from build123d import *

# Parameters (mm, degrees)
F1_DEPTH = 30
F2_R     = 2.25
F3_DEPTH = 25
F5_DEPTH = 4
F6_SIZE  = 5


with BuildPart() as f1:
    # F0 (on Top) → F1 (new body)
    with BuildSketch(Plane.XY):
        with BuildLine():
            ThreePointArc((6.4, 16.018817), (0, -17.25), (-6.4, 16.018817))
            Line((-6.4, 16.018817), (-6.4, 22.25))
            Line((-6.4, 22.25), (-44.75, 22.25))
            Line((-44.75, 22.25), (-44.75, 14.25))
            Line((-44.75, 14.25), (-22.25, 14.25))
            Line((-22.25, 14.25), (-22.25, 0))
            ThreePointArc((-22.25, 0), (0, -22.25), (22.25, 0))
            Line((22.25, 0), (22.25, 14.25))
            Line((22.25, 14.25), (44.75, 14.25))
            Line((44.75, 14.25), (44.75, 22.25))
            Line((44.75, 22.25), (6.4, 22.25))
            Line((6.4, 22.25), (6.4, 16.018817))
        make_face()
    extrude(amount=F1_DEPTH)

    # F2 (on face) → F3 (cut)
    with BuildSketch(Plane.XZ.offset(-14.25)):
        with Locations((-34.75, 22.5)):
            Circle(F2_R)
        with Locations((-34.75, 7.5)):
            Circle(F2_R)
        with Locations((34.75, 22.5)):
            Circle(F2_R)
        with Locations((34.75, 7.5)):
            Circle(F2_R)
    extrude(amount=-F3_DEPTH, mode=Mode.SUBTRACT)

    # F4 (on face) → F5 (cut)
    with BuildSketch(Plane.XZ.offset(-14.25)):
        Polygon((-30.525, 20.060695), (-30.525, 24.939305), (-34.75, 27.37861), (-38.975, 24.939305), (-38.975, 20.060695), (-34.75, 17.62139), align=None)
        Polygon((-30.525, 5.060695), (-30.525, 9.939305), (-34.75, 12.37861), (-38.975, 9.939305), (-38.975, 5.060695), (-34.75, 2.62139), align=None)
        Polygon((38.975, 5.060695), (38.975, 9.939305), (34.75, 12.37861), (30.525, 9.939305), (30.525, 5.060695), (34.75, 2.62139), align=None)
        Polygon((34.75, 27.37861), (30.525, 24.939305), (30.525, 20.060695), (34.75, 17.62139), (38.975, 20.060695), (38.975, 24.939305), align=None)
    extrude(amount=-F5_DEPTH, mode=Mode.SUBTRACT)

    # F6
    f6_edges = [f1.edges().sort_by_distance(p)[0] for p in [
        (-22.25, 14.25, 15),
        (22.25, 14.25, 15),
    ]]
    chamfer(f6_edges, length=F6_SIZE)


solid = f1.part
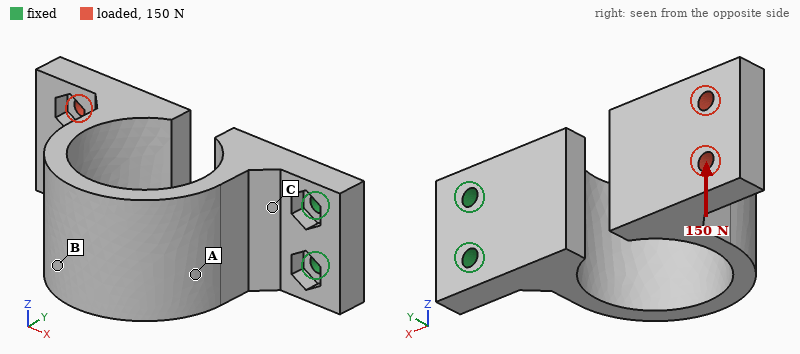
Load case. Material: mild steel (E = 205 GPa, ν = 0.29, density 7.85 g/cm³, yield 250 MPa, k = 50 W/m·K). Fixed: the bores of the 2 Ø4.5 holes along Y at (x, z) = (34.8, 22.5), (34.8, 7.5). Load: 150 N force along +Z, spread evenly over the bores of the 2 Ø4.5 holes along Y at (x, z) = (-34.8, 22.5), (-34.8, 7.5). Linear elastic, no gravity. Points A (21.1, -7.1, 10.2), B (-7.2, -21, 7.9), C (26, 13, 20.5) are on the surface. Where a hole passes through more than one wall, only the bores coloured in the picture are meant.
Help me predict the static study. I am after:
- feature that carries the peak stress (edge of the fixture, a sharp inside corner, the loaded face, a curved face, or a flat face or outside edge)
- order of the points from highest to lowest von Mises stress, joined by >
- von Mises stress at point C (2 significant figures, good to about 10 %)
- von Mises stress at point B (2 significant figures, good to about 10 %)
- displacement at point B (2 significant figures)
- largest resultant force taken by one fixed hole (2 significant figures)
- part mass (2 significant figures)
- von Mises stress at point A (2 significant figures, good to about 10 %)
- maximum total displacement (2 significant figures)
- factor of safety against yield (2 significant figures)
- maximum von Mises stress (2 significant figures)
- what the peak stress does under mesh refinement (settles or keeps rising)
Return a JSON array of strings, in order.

["a curved face", "A > B > C", "12 MPa", "29 MPa", "0.044 mm", "580 N", "260 g", "52 MPa", "0.22 mm", "3.9", "65 MPa", "settles"]
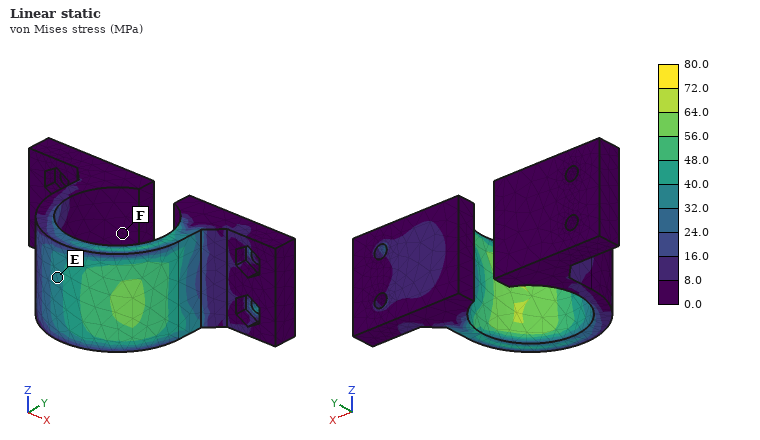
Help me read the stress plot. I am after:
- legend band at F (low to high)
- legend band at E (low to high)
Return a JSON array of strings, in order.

["0.0 to 8.0 MPa", "32.0 to 40.0 MPa"]
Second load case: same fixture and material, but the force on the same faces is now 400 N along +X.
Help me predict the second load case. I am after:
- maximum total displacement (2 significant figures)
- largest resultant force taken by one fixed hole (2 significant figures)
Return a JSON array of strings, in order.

["0.77 mm", "200 N"]
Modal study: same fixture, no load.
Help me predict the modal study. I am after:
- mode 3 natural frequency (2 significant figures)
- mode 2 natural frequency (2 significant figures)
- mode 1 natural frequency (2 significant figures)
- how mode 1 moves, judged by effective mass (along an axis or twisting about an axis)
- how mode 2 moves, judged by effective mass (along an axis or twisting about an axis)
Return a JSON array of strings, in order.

["780 Hz", "520 Hz", "360 Hz", "along Y", "along Z"]
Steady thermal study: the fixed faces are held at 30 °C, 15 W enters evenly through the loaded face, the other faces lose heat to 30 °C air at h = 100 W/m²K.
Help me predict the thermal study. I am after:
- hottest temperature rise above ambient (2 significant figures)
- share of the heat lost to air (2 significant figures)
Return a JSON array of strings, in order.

["40 K", "97 %"]
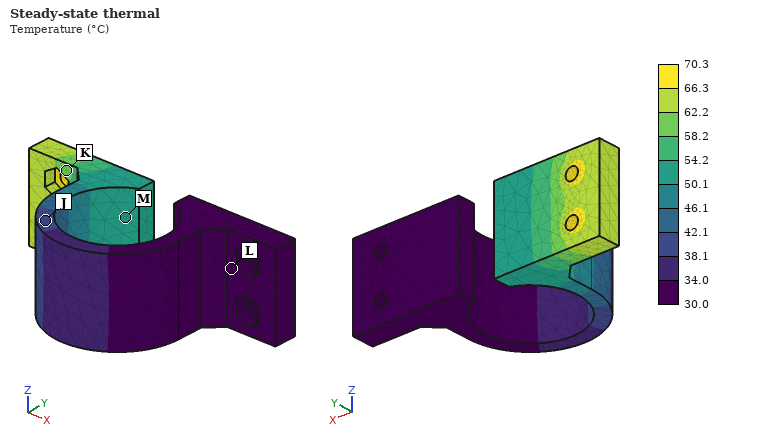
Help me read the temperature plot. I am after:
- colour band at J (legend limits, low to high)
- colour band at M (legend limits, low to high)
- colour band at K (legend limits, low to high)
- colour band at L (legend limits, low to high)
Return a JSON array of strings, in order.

["38.1 to 42.1 °C", "50.1 to 54.2 °C", "58.2 to 62.2 °C", "30.0 to 34.0 °C"]
